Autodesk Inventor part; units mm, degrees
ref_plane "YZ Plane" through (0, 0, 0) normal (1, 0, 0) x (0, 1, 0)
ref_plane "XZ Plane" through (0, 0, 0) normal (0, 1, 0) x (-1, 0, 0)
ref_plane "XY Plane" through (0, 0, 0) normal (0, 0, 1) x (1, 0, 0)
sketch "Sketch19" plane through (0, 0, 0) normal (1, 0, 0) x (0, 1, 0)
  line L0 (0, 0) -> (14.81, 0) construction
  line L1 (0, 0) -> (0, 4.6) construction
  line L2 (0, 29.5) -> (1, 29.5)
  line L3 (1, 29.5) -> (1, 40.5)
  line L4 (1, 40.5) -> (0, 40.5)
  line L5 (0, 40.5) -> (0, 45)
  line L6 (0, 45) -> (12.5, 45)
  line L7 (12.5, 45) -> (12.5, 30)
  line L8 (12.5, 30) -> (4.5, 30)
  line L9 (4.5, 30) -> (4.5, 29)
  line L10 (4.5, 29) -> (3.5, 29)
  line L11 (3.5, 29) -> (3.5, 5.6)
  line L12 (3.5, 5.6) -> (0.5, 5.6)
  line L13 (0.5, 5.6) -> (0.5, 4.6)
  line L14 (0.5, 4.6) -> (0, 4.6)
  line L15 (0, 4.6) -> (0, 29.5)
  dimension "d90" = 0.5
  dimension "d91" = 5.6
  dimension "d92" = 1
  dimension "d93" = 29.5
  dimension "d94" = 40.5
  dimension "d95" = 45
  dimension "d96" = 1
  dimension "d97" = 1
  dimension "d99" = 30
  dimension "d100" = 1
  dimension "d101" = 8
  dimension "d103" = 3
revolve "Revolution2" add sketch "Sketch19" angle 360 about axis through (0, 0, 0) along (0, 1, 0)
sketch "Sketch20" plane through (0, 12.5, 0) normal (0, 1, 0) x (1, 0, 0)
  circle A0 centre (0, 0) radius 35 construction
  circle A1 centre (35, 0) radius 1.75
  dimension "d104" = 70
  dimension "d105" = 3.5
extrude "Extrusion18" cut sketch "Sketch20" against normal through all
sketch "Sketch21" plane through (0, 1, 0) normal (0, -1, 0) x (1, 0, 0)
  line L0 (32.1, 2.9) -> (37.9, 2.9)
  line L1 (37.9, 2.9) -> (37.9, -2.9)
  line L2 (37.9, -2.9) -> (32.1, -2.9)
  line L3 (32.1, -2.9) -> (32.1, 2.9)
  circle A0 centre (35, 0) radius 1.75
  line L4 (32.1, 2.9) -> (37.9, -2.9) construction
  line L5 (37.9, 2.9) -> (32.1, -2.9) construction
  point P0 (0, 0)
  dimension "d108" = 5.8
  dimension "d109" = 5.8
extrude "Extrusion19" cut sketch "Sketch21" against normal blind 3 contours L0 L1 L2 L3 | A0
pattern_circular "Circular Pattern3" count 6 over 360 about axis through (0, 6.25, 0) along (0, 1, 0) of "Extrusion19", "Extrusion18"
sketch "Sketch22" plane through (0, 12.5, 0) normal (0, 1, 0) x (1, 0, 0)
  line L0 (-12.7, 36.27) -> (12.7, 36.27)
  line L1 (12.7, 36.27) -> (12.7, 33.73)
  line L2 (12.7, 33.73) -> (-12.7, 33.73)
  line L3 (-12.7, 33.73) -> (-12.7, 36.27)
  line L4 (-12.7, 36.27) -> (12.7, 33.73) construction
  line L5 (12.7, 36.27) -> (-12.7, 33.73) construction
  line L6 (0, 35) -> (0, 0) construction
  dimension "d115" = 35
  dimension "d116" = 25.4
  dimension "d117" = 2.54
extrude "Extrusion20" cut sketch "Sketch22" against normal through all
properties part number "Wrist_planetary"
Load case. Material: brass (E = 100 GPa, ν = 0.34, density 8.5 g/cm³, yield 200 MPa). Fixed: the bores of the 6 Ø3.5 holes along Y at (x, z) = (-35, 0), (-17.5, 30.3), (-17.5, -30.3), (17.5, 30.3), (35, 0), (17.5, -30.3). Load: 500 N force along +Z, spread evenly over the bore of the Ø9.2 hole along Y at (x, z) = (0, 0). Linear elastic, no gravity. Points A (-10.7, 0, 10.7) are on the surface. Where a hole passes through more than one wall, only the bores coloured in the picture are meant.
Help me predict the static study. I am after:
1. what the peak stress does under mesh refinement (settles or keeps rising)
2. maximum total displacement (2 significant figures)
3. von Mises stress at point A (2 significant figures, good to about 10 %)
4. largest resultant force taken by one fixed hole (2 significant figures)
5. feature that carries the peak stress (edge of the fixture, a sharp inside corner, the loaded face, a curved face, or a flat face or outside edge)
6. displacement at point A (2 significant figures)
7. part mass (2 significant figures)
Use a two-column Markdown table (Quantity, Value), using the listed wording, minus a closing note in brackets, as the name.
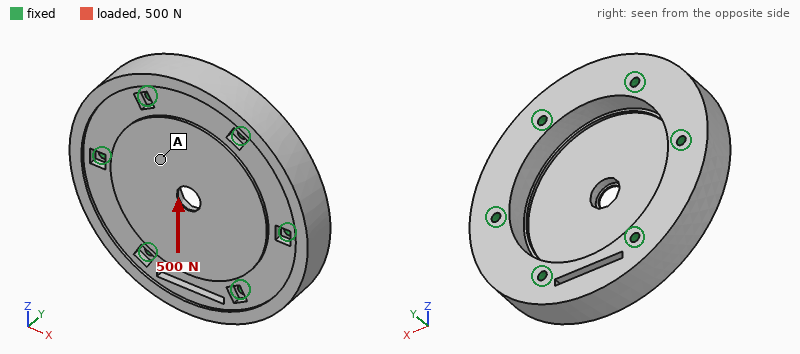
| Quantity | Value |
|---|---|
| what the peak stress does under mesh refinement | keeps rising |
| maximum total displacement | 2.1 µm |
| von Mises stress at point A | 2.8 MPa |
| largest resultant force taken by one fixed hole | 99 N |
| feature that carries the peak stress | a sharp inside corner |
| displacement at point A | 0.48 µm |
| part mass | 420 g |
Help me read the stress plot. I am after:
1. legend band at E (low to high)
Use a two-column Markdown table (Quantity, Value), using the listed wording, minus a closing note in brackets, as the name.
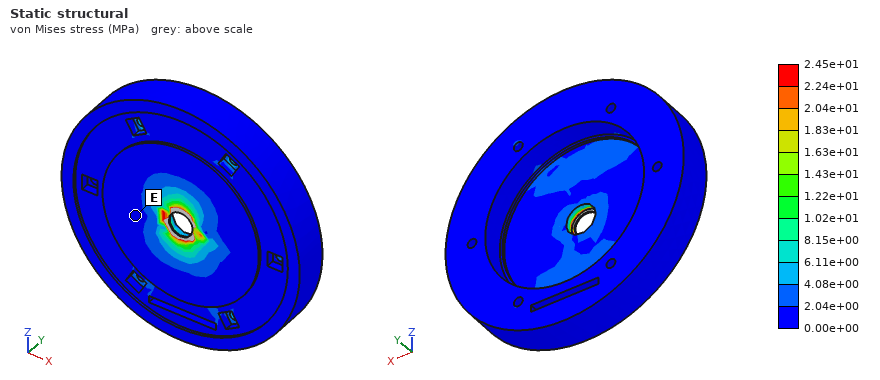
| Quantity | Value |
|---|---|
| legend band at E | 0.00e+00 to 2.04e+00 MPa |
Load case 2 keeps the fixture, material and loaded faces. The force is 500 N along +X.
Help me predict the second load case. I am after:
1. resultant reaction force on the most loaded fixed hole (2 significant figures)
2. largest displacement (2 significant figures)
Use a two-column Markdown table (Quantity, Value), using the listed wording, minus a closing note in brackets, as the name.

| Quantity | Value |
|---|---|
| resultant reaction force on the most loaded fixed hole | 110 N |
| largest displacement | 2.0 µm |
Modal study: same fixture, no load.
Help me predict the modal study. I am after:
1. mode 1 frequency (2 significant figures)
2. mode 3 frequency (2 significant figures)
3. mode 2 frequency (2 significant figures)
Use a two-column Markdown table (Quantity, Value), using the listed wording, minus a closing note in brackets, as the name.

| Quantity | Value |
|---|---|
| mode 1 frequency | 5500 Hz |
| mode 3 frequency | 10 kHz |
| mode 2 frequency | 10 kHz |
